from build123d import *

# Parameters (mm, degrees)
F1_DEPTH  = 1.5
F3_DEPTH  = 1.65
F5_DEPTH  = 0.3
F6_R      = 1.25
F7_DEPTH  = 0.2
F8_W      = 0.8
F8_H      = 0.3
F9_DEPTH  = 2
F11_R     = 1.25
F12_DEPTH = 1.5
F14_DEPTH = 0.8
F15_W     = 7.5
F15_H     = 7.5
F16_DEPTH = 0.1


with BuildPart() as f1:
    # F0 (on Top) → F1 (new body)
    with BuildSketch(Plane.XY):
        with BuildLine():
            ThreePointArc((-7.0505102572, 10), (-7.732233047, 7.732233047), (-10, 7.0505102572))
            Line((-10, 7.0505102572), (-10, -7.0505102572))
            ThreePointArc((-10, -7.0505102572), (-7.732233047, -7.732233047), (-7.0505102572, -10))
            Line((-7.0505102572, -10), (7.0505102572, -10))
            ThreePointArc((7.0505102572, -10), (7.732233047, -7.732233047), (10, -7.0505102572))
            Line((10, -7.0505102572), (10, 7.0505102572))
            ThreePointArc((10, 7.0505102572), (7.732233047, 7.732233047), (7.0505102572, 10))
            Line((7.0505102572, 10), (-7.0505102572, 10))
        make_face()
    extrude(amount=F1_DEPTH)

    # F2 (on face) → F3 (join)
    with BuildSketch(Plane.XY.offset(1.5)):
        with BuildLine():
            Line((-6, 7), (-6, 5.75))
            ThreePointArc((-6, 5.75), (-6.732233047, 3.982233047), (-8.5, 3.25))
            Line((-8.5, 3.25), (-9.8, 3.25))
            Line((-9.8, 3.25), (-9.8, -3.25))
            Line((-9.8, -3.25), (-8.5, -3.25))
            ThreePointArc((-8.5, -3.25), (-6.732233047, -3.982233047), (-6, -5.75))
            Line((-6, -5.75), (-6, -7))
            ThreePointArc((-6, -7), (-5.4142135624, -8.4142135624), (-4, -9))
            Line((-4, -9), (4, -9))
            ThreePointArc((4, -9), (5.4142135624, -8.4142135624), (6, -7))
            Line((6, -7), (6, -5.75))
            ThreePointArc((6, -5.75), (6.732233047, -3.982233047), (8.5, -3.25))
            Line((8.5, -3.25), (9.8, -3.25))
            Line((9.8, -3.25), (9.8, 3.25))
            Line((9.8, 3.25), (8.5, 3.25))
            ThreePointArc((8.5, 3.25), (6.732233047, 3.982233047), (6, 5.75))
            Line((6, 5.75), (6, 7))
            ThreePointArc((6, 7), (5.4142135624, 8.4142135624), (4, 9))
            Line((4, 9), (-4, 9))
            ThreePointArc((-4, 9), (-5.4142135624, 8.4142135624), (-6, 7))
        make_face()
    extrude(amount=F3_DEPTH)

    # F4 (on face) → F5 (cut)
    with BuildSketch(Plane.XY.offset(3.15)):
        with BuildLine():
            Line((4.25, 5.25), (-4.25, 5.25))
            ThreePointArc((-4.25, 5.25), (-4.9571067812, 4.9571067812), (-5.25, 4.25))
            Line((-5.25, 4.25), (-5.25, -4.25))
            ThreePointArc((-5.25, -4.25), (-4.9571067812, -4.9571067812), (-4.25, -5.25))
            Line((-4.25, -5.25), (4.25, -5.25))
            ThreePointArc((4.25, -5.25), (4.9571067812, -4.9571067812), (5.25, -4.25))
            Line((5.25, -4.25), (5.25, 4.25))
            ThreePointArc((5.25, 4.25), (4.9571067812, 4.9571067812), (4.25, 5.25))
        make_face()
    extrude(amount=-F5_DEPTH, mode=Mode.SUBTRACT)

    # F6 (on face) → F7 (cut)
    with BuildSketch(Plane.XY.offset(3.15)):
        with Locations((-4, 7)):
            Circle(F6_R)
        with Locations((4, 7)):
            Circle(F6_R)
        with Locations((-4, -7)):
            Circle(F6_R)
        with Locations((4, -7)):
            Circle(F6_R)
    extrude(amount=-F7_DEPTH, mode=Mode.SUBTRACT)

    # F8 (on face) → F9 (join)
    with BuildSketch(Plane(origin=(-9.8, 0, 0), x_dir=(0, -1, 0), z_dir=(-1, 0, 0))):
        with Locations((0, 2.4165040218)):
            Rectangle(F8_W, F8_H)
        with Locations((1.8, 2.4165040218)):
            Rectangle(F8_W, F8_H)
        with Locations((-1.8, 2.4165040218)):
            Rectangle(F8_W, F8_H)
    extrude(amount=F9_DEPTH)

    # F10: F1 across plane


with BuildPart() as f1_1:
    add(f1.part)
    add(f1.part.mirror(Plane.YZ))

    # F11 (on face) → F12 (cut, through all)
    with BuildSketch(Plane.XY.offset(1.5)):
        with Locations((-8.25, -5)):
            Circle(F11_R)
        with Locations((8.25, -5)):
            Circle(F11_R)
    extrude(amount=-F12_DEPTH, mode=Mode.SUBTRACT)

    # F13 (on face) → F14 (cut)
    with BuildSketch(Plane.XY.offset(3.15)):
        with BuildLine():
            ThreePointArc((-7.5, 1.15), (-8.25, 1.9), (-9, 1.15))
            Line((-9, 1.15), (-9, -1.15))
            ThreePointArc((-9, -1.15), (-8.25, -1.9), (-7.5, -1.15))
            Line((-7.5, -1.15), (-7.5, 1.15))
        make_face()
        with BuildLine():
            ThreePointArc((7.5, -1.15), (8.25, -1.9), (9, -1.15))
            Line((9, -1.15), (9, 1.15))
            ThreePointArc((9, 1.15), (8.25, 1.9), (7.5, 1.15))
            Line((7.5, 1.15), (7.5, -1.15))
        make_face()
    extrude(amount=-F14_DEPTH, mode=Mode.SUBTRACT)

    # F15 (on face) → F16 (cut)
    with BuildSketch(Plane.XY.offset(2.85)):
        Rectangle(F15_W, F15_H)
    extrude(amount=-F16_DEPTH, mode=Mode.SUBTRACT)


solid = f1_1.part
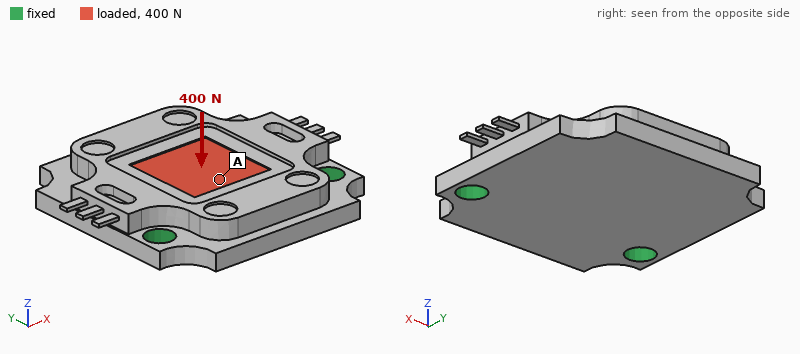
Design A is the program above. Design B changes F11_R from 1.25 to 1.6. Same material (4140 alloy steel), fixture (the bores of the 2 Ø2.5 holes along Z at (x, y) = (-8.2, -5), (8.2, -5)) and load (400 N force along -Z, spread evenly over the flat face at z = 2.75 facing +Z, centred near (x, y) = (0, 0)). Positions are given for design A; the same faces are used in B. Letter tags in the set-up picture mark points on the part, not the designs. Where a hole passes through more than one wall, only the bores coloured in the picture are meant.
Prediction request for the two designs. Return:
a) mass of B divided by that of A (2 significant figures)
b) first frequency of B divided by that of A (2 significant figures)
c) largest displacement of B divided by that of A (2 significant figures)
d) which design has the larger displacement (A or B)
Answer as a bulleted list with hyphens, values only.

- 0.99
- 1.2
- 0.74
- A
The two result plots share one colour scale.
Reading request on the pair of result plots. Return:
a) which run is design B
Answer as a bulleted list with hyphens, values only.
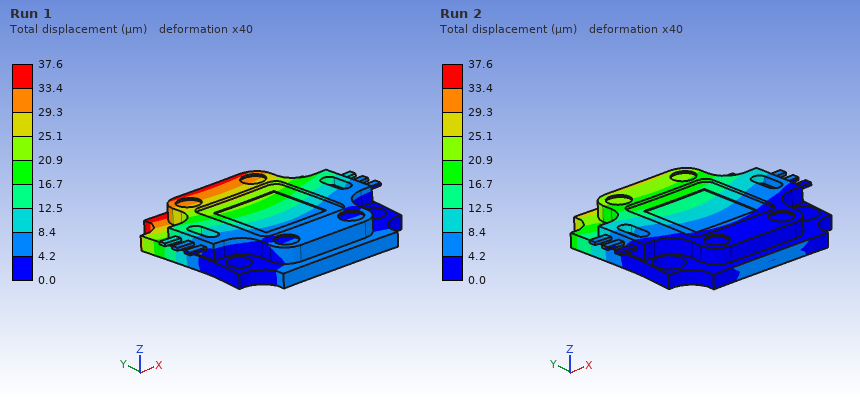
- Run 2
